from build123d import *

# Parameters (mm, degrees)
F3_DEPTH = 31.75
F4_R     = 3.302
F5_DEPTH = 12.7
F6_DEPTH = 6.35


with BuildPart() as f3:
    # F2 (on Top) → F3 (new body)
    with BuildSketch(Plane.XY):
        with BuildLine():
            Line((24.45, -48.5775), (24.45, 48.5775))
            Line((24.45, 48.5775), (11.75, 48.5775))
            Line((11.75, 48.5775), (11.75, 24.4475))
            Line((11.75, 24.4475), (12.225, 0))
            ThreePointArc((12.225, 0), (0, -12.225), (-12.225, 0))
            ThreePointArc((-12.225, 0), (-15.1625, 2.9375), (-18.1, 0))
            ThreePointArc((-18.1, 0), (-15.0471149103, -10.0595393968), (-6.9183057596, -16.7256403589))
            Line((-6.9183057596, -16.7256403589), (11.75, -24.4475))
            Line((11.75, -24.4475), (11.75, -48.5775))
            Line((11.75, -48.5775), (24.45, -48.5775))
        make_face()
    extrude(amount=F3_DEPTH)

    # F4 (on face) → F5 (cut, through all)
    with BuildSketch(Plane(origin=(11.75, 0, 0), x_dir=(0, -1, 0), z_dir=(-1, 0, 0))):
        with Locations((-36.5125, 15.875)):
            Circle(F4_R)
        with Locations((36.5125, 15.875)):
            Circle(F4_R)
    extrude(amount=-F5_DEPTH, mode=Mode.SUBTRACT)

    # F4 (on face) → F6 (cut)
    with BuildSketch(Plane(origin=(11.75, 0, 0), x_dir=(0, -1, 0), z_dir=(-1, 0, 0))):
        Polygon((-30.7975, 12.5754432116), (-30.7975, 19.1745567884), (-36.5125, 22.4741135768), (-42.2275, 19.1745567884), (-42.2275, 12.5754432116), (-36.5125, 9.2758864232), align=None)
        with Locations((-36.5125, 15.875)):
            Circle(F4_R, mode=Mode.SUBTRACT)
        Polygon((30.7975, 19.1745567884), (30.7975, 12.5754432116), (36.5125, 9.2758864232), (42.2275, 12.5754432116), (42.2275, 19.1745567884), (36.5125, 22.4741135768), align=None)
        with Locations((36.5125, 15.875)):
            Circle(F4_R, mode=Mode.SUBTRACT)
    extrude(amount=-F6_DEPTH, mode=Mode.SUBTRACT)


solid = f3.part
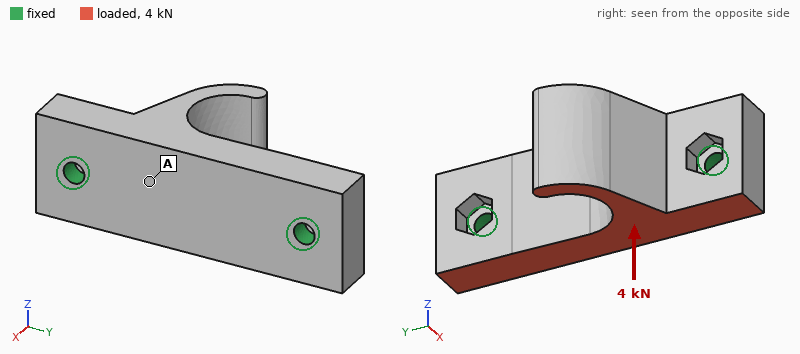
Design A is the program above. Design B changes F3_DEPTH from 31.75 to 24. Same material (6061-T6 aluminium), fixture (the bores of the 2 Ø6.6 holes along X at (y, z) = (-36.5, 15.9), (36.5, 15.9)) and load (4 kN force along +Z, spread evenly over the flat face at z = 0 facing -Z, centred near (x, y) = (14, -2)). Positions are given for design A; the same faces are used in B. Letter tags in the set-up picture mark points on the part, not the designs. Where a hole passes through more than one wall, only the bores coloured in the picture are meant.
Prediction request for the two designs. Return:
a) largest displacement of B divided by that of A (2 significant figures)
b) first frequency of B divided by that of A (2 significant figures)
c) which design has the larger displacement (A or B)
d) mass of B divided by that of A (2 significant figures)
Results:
1.3
1.0
B
0.75
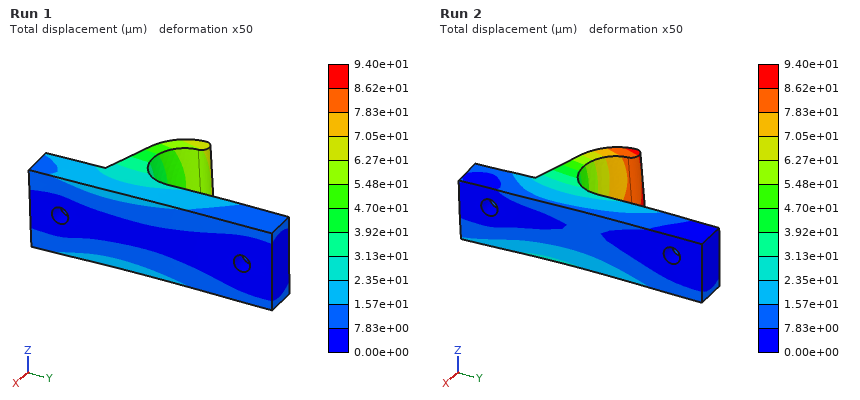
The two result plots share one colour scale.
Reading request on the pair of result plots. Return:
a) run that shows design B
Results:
Run 2
